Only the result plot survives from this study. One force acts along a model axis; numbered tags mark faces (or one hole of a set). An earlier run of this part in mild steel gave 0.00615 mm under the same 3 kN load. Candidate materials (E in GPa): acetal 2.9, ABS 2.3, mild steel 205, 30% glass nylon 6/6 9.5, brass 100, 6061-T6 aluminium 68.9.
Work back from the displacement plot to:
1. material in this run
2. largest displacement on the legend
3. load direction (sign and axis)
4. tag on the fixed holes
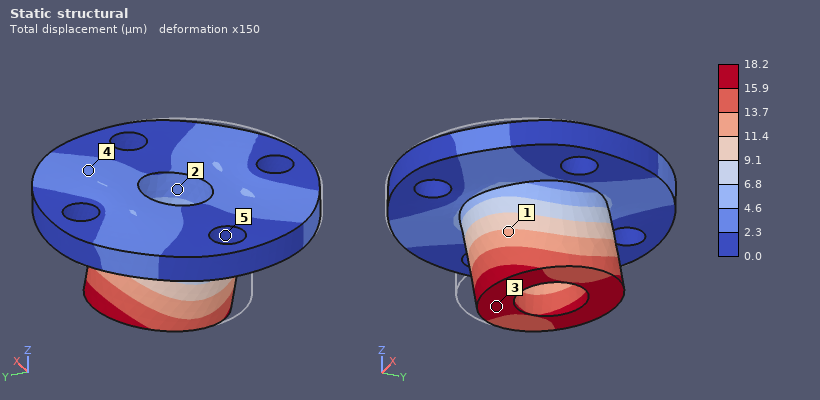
6061-T6 aluminium
18.2 µm
+Y
5
